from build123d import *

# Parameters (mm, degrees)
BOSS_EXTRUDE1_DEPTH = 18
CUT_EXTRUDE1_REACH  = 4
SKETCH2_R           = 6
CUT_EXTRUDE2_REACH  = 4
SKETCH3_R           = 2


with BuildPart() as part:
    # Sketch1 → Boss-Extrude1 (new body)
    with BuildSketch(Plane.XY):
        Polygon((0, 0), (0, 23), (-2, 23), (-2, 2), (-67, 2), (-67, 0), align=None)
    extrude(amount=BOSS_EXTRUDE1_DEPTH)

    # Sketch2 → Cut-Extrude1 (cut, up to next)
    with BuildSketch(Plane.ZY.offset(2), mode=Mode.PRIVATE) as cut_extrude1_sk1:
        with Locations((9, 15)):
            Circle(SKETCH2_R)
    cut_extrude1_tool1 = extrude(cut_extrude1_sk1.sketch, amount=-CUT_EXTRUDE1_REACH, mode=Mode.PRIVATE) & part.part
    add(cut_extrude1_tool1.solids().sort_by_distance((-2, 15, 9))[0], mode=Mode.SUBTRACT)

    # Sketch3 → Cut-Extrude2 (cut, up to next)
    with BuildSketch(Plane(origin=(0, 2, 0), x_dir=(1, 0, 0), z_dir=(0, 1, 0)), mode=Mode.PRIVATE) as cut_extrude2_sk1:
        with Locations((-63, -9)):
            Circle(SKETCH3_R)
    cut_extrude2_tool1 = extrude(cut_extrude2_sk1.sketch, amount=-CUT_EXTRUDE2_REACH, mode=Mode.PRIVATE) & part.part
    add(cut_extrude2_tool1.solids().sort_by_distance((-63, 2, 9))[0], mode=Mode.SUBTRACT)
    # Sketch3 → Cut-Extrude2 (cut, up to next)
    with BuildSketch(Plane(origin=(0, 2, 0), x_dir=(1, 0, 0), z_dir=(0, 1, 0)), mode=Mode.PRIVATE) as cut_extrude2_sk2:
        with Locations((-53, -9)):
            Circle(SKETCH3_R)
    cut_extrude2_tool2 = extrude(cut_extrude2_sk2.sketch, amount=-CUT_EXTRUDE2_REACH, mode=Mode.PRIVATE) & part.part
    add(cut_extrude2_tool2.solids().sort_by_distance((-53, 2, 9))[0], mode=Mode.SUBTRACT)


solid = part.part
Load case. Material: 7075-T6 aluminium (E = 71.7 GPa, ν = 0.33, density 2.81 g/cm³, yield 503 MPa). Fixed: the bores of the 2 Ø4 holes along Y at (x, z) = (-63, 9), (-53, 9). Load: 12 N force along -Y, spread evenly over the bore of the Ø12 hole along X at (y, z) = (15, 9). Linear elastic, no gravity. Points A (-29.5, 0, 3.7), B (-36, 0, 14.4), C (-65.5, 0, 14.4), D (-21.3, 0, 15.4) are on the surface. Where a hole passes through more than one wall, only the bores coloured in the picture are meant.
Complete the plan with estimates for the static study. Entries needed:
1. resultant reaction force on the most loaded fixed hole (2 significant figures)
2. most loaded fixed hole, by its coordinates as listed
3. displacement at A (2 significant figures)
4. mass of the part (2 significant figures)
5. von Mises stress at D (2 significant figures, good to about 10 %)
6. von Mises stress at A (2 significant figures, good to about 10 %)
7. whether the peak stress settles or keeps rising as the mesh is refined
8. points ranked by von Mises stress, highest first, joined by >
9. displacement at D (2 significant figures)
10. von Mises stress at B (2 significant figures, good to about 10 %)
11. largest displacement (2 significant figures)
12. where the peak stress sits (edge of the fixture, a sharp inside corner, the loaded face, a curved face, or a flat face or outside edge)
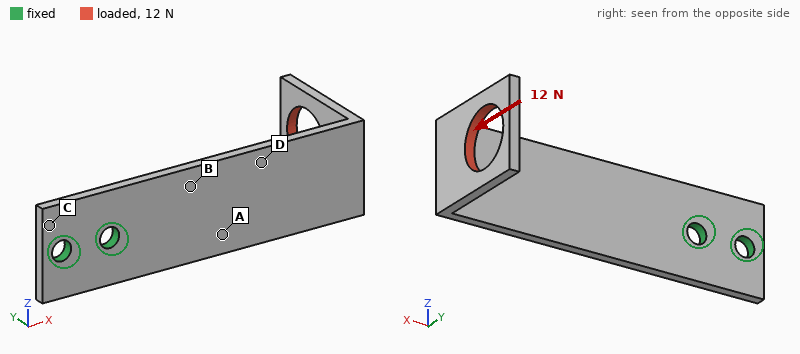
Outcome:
25 N
(-53, 9)
0.15 mm
8.1 g
20 MPa
28 MPa
keeps rising
B > A > D > C
0.27 mm
34 MPa
0.75 mm
edge of the fixture
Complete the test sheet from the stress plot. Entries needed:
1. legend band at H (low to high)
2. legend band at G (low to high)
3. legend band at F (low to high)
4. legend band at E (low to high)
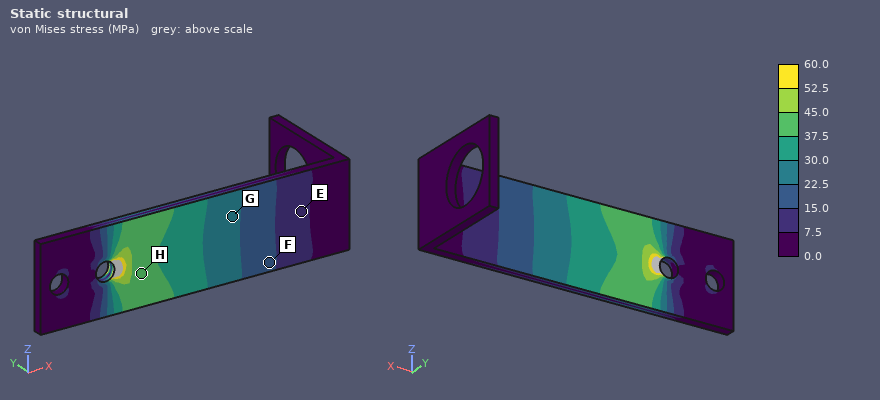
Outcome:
37.5 to 45.0 MPa
22.5 to 30.0 MPa
15.0 to 22.5 MPa
7.5 to 15.0 MPa
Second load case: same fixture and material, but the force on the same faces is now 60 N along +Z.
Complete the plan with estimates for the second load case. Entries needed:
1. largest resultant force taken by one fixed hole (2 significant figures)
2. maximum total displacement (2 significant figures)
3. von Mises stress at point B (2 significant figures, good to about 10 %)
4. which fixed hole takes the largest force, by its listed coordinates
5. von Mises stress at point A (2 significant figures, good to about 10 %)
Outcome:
240 N
0.86 mm
62 MPa
(-53, 9)
62 MPa
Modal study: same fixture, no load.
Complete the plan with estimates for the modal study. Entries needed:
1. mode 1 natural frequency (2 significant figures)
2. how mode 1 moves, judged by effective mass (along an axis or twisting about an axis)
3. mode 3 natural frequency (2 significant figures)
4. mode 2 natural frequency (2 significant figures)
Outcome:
410 Hz
along Y
1900 Hz
1300 Hz
